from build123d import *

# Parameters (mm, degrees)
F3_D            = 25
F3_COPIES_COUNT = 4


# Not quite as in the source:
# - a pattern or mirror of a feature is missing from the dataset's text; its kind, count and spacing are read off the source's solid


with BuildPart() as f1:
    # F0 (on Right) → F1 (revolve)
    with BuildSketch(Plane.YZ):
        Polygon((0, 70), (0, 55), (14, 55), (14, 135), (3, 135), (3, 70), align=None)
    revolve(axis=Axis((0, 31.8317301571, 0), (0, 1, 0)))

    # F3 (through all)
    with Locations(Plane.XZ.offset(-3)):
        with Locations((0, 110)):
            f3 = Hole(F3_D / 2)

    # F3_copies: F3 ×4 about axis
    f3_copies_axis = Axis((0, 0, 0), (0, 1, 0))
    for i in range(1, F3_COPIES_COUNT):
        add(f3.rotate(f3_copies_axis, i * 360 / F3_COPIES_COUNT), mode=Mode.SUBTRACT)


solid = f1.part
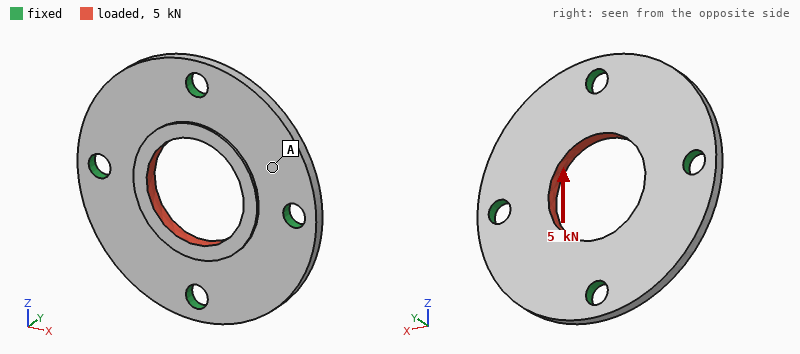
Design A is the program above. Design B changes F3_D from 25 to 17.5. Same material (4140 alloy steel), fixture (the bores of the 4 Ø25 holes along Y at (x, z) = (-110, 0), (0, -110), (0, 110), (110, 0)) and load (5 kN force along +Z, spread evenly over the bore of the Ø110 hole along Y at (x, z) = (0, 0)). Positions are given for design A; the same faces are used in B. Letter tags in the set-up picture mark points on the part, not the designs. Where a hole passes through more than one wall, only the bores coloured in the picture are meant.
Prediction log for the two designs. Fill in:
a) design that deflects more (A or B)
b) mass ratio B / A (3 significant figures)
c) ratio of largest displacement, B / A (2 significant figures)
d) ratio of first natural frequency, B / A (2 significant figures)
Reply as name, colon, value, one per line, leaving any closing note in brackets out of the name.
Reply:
design that deflects more: B
mass ratio B / A: 1.02
ratio of largest displacement, B / A: 1.1
ratio of first natural frequency, B / A: 0.88
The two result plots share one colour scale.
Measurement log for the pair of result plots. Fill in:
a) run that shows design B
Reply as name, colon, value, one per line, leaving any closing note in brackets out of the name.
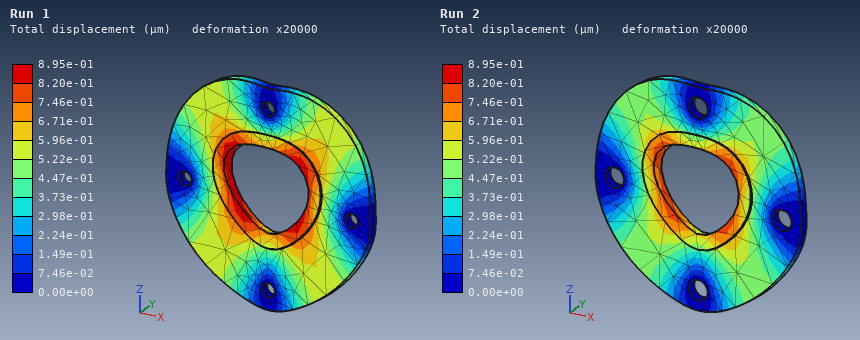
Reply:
run that shows design B: Run 1
